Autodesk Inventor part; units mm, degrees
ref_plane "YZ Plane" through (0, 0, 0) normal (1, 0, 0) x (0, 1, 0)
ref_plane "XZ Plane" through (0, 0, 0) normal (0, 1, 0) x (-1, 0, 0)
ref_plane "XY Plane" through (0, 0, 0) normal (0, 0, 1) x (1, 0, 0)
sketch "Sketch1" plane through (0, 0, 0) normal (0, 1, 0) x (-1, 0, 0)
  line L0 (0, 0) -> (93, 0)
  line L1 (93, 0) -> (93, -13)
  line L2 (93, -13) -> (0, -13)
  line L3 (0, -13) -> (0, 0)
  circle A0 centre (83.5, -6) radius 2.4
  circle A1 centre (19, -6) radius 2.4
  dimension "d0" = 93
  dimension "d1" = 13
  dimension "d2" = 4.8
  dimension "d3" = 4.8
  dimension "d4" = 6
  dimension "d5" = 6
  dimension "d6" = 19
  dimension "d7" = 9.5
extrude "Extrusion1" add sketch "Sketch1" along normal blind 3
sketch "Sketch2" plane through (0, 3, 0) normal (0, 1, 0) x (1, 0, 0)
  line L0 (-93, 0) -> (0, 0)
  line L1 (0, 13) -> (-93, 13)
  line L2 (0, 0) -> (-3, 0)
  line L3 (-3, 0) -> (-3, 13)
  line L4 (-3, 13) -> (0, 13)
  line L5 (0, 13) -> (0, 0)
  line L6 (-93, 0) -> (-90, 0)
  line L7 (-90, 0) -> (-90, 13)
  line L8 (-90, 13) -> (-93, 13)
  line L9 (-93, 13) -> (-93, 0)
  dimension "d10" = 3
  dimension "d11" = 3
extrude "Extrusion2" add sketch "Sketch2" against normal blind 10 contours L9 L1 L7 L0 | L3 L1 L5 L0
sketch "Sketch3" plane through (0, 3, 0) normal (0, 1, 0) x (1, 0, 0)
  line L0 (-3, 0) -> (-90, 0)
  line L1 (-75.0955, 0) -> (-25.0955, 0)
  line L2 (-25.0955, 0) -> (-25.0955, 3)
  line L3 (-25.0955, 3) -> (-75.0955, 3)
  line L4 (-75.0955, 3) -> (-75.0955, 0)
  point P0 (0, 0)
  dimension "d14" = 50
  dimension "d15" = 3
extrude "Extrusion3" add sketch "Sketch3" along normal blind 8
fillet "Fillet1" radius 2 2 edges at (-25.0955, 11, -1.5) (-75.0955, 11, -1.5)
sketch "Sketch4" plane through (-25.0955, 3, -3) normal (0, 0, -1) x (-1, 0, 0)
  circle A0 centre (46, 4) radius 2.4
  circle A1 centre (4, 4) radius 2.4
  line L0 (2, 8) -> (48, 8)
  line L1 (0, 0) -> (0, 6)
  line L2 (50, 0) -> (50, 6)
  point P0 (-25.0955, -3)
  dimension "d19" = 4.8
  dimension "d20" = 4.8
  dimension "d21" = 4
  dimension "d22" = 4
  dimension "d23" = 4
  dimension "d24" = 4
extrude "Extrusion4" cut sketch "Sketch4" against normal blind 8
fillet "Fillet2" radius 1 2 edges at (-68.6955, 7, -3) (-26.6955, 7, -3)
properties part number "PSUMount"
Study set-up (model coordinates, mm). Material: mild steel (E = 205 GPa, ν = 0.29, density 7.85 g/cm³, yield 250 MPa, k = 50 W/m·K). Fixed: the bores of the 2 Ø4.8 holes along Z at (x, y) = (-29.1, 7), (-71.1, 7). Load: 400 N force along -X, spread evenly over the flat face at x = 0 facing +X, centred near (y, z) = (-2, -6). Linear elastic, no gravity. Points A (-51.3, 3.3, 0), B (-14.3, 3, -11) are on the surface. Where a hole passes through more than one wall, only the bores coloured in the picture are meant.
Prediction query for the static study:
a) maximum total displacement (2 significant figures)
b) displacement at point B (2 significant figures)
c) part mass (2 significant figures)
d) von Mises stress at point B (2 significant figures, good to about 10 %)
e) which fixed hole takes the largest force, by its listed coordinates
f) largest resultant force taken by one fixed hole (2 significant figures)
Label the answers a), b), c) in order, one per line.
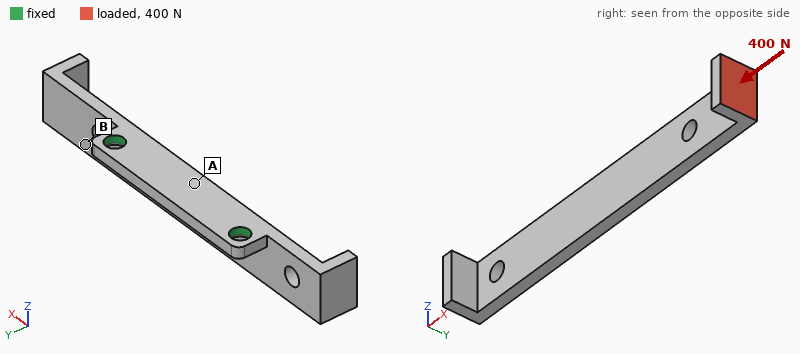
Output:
a) 0.14 mm
b) 0.033 mm
c) 40 g
d) 68 MPa
e) (-29.1, 7)
f) 230 N
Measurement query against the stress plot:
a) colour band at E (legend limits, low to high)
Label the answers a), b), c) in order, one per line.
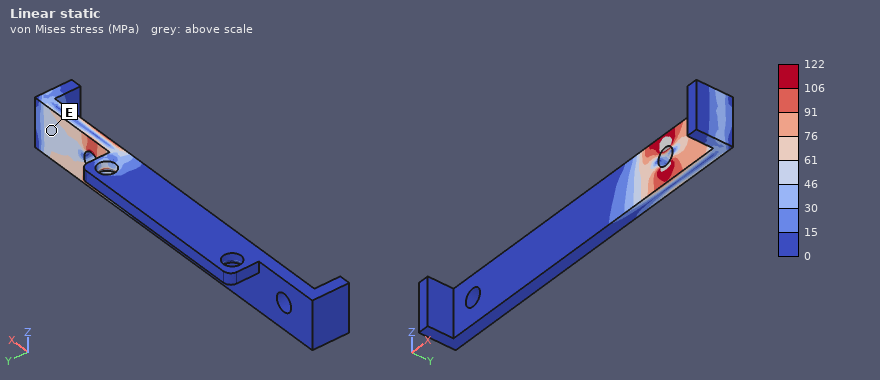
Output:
a) 46 to 61 MPa
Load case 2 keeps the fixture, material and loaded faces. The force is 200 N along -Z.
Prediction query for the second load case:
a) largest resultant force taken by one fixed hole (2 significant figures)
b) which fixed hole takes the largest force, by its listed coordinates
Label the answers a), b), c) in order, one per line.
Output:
a) 390 N
b) (-29.1, 7)
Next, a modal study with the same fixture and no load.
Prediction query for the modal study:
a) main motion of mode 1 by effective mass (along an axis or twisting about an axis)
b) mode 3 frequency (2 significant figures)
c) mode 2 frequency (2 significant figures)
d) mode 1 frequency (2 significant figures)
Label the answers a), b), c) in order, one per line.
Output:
a) along Y
b) 4600 Hz
c) 3100 Hz
d) 1900 Hz
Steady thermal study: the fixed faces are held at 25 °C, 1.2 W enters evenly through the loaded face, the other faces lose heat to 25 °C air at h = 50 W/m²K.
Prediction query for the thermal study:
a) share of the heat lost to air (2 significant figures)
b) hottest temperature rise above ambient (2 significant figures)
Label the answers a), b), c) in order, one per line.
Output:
a) 46 %
b) 16 K
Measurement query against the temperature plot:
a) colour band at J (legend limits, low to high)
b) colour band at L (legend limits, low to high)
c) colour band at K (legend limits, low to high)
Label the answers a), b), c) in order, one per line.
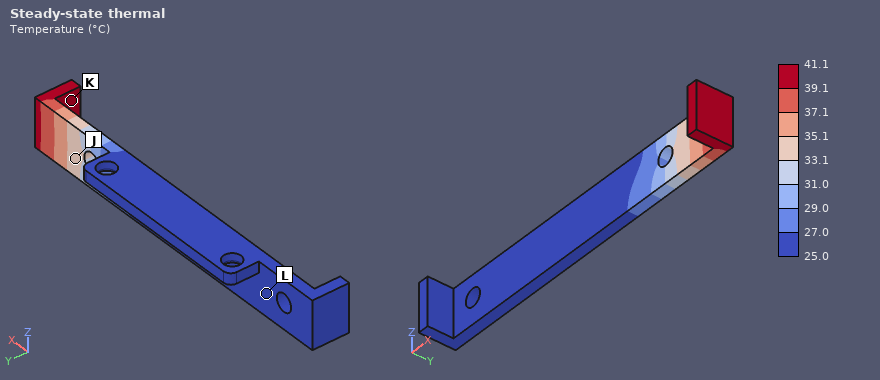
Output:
a) 33.1 to 35.1 °C
b) 25.0 to 27.0 °C
c) 39.1 to 41.1 °C
